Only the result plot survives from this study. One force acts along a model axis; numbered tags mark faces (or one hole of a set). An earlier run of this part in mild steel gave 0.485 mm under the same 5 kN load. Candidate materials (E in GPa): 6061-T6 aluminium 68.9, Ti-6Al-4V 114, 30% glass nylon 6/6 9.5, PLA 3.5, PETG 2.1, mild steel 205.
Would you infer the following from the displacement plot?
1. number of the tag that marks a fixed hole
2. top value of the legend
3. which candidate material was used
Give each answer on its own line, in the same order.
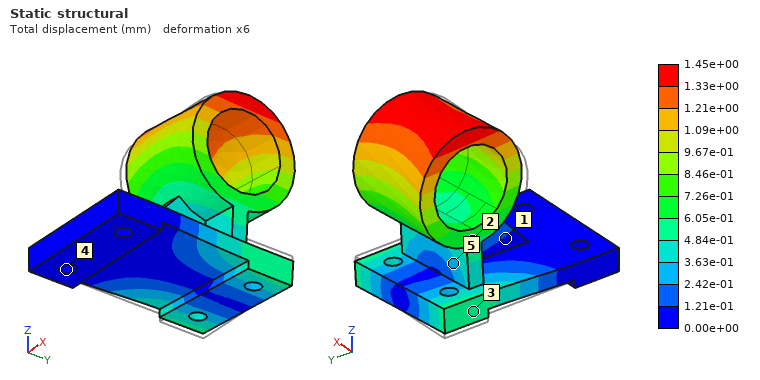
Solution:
4
1.45e+00 mm
6061-T6 aluminium
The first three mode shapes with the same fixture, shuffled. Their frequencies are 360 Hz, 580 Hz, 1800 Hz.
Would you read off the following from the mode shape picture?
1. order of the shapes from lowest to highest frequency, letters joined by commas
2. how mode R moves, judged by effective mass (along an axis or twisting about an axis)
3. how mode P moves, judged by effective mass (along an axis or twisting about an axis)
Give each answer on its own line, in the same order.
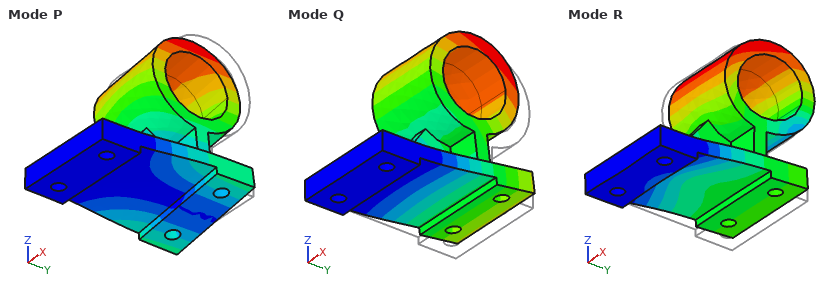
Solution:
Q, P, R
along Z
along X
